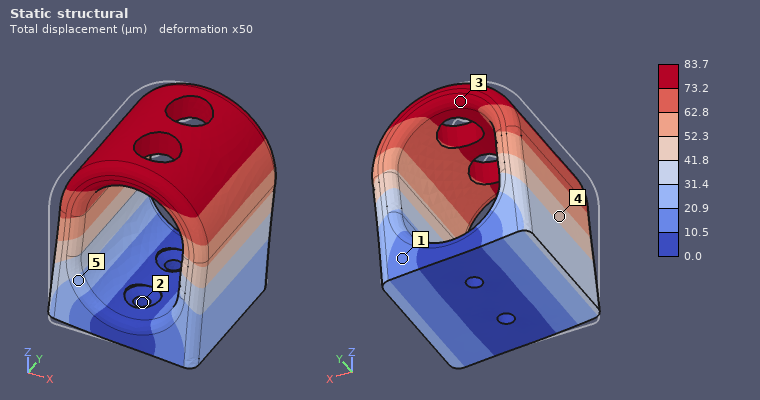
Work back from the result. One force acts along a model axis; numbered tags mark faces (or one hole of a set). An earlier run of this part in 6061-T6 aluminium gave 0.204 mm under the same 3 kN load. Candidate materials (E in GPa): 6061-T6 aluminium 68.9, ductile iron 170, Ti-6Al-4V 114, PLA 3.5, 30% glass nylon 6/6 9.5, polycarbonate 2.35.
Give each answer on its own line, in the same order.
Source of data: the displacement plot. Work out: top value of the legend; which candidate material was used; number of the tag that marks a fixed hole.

83.7 µm
ductile iron
2
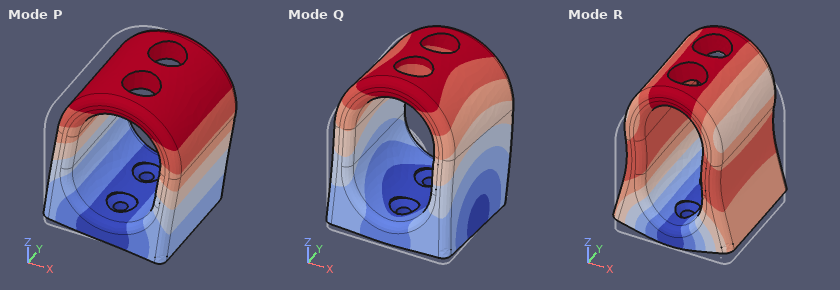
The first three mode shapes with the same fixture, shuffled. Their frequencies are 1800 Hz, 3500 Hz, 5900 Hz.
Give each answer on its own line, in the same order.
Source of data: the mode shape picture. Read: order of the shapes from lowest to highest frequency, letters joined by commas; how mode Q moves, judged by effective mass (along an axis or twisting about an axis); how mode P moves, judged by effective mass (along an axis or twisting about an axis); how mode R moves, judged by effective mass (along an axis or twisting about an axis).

P, Q, R
along Y
along X
along Z
